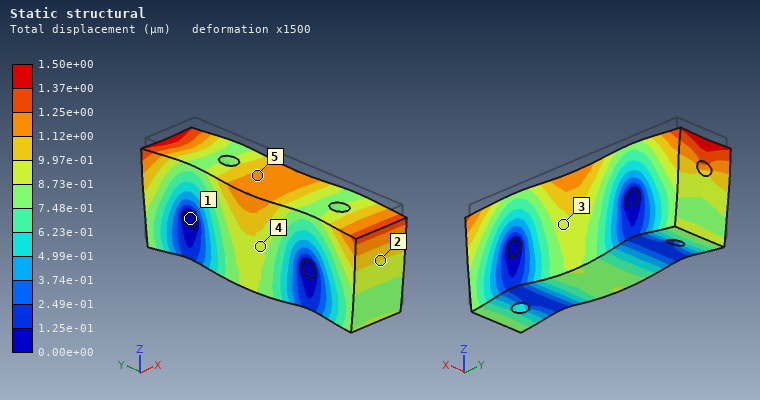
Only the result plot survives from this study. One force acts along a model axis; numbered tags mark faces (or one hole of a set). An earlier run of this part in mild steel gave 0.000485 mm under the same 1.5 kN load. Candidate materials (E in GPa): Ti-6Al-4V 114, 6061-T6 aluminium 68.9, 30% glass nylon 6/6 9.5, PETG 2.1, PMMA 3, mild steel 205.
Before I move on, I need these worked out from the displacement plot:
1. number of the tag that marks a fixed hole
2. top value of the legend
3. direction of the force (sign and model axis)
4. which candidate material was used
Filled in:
1
1.50e+00 µm
-Z
6061-T6 aluminium
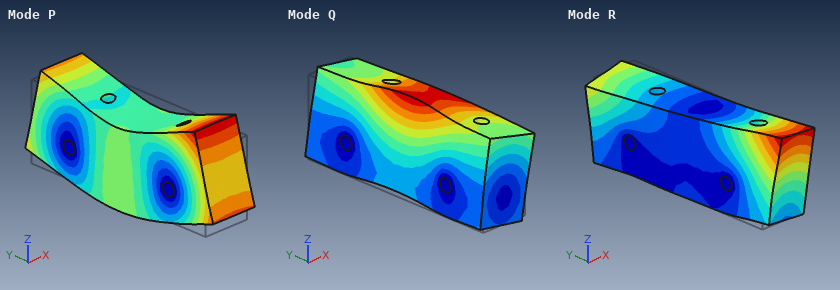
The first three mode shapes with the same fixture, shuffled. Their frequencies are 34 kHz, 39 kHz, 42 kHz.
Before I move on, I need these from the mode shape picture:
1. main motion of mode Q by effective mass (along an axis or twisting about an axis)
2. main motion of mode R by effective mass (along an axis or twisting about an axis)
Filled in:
along X
twisting about Z
